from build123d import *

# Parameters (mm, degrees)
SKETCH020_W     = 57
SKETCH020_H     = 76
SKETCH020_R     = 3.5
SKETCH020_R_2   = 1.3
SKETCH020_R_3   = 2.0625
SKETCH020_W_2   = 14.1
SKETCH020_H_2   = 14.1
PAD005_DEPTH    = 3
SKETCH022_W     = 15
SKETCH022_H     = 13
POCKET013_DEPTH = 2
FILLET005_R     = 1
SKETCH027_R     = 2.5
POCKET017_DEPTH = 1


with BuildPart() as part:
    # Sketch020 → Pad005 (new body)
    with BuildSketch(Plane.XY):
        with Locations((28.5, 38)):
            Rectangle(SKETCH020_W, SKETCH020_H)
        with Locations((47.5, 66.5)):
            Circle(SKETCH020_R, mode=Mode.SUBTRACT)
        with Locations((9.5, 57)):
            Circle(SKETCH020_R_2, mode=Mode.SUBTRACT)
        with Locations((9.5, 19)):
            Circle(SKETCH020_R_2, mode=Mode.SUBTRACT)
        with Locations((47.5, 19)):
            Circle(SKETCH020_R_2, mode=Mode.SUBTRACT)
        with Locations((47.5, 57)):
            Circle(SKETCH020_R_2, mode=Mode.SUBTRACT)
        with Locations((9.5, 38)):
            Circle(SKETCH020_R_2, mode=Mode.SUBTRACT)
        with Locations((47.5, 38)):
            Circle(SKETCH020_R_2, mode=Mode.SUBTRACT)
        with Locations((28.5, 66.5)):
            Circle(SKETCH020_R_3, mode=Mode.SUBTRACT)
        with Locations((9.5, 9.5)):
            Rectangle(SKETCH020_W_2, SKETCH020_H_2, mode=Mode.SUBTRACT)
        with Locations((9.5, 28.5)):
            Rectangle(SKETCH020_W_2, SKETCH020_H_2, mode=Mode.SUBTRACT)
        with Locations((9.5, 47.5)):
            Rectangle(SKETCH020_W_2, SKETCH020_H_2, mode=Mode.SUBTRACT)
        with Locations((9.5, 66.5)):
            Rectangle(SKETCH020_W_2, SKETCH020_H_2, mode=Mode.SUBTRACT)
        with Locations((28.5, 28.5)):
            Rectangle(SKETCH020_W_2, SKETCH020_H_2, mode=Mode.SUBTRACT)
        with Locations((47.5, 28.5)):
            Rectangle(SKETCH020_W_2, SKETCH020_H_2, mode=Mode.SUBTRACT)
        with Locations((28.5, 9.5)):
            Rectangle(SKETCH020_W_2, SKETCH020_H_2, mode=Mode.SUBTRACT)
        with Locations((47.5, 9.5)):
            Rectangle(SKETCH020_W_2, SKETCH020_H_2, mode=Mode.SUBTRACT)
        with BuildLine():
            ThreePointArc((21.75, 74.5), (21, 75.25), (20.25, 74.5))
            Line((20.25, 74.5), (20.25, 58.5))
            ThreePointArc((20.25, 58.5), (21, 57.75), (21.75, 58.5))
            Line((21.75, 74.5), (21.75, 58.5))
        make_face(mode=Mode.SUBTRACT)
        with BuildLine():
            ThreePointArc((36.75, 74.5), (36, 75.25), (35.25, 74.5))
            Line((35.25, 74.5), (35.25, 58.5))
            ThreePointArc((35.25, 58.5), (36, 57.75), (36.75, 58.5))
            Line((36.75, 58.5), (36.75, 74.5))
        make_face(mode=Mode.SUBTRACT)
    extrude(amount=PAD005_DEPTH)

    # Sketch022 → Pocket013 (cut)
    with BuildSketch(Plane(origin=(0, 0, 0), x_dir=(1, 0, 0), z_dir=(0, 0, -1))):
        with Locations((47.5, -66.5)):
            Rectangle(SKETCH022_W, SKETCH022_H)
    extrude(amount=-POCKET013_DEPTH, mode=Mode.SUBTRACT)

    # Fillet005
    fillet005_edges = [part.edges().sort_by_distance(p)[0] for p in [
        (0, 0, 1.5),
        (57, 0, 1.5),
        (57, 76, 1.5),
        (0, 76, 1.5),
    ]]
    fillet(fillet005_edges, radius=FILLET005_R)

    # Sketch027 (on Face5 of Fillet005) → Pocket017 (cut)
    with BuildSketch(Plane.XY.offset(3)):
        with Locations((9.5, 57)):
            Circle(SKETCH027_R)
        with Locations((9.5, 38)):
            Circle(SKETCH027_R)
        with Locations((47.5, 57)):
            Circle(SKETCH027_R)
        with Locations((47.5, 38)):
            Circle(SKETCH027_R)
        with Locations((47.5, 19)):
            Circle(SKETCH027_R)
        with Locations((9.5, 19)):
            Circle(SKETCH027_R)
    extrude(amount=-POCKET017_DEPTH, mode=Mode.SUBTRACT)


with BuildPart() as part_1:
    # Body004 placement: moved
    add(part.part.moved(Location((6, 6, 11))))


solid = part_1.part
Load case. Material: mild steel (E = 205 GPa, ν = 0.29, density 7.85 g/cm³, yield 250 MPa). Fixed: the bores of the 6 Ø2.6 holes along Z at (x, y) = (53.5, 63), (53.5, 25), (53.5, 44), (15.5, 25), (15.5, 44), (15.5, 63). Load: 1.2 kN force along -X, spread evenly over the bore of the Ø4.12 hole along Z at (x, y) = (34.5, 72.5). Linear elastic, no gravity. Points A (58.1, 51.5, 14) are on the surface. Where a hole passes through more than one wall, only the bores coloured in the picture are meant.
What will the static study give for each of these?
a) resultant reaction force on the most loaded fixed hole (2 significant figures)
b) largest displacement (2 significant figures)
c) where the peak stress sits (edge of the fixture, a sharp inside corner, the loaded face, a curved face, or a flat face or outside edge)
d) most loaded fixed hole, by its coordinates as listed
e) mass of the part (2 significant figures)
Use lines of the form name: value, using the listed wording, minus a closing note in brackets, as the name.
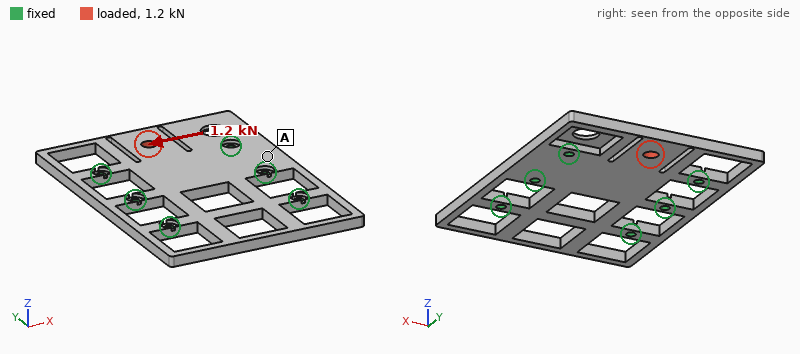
resultant reaction force on the most loaded fixed hole: 790 N
largest displacement: 13 µm
where the peak stress sits: a curved face
most loaded fixed hole, by its coordinates as listed: (53.5, 63)
mass of the part: 58 g
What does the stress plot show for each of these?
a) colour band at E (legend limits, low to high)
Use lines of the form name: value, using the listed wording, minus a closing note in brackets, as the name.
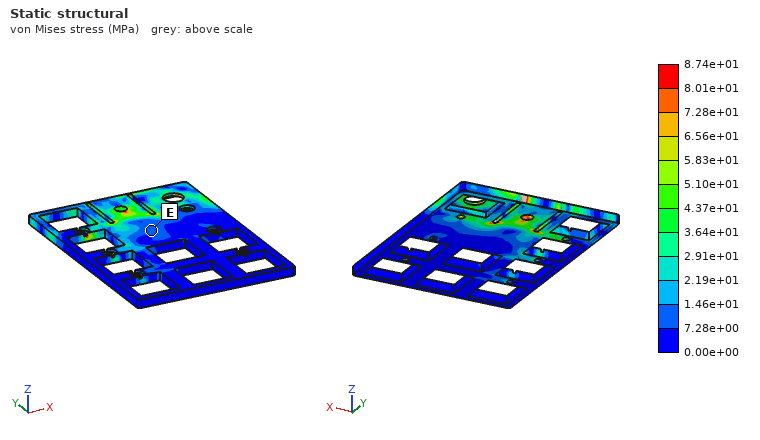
colour band at E: 7.28e+00 to 1.46e+01 MPa
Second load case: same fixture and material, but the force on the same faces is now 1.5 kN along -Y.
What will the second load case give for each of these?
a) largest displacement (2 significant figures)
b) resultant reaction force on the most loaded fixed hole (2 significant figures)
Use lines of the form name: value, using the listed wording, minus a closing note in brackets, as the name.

largest displacement: 7.7 µm
resultant reaction force on the most loaded fixed hole: 660 N
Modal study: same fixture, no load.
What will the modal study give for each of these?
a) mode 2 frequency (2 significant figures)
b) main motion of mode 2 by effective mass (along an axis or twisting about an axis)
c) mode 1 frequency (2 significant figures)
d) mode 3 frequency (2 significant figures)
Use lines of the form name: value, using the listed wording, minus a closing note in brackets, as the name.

mode 2 frequency: 3500 Hz
main motion of mode 2 by effective mass: along Z
mode 1 frequency: 3400 Hz
mode 3 frequency: 4800 Hz
